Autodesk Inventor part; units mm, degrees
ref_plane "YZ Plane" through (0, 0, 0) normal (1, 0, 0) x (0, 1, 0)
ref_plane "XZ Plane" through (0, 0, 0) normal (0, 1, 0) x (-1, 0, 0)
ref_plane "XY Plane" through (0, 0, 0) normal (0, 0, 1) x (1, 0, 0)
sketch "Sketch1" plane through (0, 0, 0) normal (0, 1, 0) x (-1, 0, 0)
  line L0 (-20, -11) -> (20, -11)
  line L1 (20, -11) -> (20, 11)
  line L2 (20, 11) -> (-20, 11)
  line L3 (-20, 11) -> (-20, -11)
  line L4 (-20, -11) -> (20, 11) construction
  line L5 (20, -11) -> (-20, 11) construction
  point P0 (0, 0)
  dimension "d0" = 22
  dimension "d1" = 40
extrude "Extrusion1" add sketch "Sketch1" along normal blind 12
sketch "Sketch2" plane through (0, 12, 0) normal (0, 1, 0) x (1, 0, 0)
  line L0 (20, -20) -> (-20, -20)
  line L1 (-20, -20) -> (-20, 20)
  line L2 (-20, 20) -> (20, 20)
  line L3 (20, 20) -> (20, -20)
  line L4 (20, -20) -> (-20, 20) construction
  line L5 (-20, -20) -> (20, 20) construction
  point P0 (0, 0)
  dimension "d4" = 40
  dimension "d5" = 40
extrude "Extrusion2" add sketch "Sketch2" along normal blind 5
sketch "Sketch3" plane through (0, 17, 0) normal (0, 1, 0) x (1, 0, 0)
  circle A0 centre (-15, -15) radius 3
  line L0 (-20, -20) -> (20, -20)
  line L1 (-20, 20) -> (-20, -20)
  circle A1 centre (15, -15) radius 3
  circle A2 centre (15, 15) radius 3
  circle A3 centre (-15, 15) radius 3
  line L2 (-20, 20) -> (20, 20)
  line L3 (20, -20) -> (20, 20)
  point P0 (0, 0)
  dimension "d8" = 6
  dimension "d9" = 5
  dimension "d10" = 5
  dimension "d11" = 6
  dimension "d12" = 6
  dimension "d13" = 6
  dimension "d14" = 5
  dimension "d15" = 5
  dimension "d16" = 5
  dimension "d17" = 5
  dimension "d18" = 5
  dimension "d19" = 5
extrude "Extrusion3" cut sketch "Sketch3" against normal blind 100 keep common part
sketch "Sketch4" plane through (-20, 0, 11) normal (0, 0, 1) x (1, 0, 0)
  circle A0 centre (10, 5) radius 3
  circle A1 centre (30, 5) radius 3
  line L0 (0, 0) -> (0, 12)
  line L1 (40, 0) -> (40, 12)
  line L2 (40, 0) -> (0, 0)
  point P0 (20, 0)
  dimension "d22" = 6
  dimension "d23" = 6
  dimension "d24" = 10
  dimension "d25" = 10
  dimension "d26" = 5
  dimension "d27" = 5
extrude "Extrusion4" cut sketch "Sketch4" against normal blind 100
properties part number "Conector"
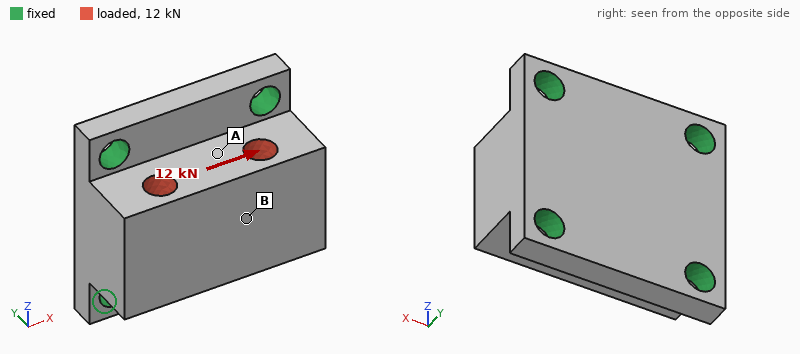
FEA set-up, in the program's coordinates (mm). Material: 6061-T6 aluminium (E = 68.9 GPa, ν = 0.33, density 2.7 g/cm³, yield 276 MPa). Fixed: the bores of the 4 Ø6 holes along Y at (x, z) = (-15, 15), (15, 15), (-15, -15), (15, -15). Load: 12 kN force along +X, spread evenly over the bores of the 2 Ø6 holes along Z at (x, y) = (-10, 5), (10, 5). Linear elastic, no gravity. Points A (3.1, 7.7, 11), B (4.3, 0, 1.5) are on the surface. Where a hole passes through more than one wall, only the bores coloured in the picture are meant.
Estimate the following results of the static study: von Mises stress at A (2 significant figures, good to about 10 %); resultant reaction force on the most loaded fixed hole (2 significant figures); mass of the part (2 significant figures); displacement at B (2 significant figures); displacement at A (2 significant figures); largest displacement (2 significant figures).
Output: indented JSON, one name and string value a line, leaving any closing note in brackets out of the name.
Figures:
{
  "von Mises stress at A": "35 MPa",
  "resultant reaction force on the most loaded fixed hole": "3.8 kN",
  "mass of the part": "45 g",
  "displacement at B": "23 µm",
  "displacement at A": "14 µm",
  "largest displacement": "28 µm"
}
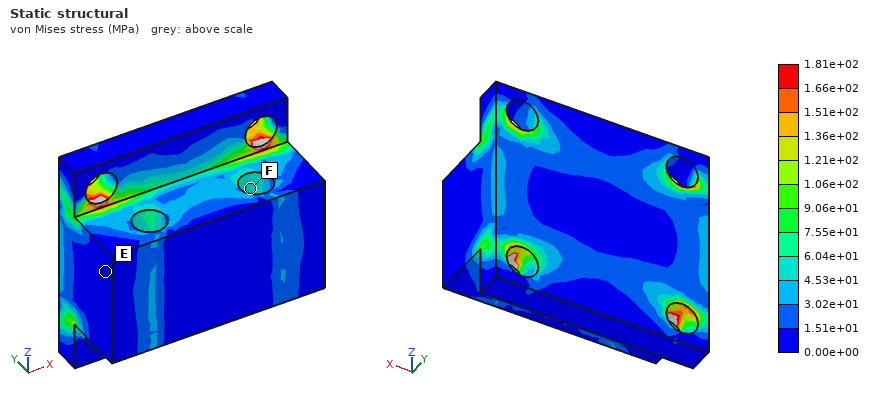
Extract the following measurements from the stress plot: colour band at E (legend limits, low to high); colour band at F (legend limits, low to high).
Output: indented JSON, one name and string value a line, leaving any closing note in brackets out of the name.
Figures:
{
  "colour band at E": "0.00e+00 to 1.51e+01 MPa",
  "colour band at F": "4.53e+01 to 6.04e+01 MPa"
}
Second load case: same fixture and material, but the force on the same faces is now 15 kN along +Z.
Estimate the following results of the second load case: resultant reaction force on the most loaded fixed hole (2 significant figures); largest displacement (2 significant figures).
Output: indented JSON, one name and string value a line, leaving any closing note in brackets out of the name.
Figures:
{
  "resultant reaction force on the most loaded fixed hole": "4.8 kN",
  "largest displacement": "29 µm"
}
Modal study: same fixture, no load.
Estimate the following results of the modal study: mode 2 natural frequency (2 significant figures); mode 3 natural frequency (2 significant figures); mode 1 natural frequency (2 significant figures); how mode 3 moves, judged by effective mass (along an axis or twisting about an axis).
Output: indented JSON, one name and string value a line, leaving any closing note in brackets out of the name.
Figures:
{
  "mode 2 natural frequency": "23 kHz",
  "mode 3 natural frequency": "26 kHz",
  "mode 1 natural frequency": "23 kHz",
  "how mode 3 moves, judged by effective mass": "along Z"
}
